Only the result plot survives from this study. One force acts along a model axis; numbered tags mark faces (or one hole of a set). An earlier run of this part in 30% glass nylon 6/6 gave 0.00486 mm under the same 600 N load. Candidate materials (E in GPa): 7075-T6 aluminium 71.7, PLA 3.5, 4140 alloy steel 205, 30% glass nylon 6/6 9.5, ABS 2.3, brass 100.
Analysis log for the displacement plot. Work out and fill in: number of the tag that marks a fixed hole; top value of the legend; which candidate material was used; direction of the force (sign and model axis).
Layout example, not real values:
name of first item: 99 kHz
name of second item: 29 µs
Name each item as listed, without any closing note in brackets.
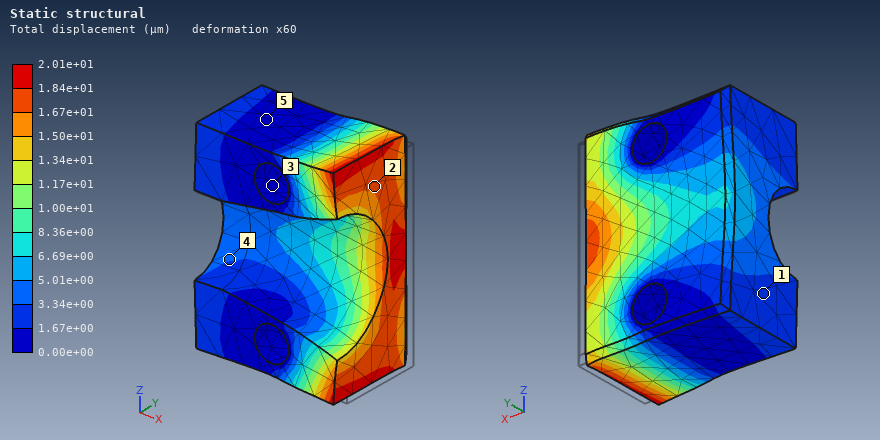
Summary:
number of the tag that marks a fixed hole: 3
top value of the legend: 2.01e+01 µm
which candidate material was used: ABS
direction of the force: -X
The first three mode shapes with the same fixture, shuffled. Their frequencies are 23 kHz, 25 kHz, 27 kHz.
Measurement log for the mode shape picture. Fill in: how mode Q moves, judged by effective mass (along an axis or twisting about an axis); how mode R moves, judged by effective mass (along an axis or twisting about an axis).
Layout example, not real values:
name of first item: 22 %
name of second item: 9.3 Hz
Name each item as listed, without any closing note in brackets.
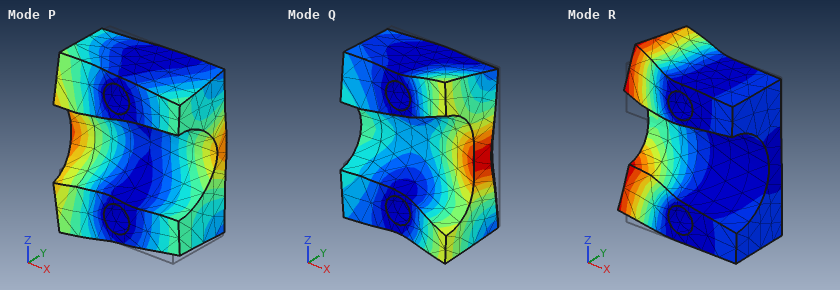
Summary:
how mode Q moves, judged by effective mass: along Y
how mode R moves, judged by effective mass: along Z
